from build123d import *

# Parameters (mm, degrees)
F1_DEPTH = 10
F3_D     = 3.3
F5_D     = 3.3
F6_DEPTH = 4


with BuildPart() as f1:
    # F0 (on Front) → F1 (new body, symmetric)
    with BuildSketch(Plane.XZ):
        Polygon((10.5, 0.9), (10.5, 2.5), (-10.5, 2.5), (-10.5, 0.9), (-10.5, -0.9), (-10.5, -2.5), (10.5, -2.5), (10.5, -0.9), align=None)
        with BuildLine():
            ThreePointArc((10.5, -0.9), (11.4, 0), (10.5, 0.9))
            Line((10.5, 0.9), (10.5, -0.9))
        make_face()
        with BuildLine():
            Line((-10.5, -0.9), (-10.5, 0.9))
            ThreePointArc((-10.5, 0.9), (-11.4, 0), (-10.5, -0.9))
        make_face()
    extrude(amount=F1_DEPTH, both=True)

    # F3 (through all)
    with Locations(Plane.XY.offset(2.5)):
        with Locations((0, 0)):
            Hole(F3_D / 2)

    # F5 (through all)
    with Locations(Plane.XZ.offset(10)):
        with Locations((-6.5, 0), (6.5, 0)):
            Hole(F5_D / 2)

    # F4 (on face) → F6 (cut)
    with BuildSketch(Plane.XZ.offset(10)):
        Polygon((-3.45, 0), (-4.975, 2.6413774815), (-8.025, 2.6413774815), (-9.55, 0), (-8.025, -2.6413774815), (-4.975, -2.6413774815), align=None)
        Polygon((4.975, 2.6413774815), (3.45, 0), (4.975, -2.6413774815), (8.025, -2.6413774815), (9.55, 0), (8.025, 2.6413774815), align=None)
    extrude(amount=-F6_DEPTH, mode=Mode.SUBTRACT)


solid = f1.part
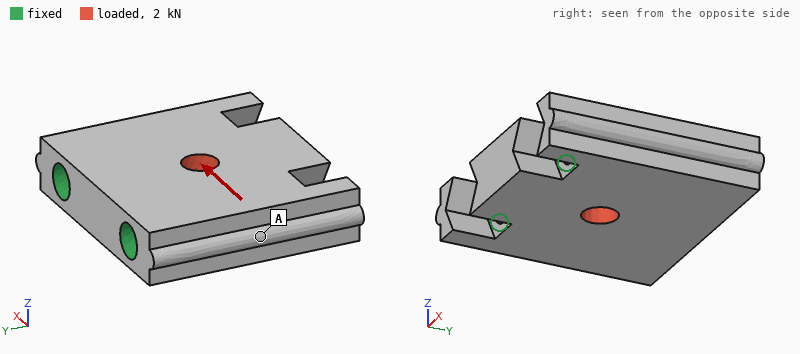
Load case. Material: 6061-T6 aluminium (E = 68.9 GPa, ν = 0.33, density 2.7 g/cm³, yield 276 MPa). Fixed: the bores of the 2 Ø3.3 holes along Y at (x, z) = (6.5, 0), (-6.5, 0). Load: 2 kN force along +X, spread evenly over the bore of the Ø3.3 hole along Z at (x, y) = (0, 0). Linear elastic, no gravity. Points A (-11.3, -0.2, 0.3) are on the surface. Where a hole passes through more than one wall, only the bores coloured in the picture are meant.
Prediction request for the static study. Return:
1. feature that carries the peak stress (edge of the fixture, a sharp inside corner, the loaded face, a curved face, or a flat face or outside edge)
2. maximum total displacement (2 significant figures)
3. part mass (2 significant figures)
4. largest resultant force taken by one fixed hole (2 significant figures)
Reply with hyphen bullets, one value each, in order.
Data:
- the loaded face
- 2.0 µm
- 4.5 g
- 1.0 kN
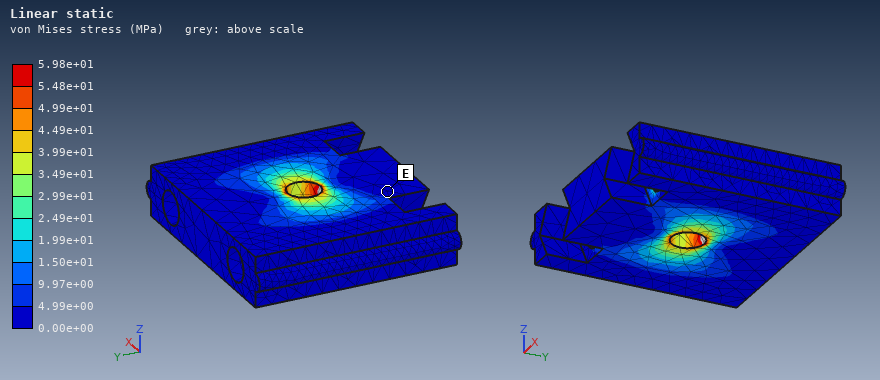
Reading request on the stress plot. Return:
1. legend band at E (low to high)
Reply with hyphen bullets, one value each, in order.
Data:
- 0.00e+00 to 4.99e+00 MPa
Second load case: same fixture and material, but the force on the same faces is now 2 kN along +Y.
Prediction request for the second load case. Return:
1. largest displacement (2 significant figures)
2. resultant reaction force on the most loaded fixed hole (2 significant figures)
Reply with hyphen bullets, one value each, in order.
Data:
- 3.3 µm
- 1.0 kN
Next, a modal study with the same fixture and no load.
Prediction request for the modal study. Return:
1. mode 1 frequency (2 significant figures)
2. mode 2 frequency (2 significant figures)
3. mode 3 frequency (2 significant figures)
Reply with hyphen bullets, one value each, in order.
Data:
- 57 kHz
- 62 kHz
- 62 kHz
